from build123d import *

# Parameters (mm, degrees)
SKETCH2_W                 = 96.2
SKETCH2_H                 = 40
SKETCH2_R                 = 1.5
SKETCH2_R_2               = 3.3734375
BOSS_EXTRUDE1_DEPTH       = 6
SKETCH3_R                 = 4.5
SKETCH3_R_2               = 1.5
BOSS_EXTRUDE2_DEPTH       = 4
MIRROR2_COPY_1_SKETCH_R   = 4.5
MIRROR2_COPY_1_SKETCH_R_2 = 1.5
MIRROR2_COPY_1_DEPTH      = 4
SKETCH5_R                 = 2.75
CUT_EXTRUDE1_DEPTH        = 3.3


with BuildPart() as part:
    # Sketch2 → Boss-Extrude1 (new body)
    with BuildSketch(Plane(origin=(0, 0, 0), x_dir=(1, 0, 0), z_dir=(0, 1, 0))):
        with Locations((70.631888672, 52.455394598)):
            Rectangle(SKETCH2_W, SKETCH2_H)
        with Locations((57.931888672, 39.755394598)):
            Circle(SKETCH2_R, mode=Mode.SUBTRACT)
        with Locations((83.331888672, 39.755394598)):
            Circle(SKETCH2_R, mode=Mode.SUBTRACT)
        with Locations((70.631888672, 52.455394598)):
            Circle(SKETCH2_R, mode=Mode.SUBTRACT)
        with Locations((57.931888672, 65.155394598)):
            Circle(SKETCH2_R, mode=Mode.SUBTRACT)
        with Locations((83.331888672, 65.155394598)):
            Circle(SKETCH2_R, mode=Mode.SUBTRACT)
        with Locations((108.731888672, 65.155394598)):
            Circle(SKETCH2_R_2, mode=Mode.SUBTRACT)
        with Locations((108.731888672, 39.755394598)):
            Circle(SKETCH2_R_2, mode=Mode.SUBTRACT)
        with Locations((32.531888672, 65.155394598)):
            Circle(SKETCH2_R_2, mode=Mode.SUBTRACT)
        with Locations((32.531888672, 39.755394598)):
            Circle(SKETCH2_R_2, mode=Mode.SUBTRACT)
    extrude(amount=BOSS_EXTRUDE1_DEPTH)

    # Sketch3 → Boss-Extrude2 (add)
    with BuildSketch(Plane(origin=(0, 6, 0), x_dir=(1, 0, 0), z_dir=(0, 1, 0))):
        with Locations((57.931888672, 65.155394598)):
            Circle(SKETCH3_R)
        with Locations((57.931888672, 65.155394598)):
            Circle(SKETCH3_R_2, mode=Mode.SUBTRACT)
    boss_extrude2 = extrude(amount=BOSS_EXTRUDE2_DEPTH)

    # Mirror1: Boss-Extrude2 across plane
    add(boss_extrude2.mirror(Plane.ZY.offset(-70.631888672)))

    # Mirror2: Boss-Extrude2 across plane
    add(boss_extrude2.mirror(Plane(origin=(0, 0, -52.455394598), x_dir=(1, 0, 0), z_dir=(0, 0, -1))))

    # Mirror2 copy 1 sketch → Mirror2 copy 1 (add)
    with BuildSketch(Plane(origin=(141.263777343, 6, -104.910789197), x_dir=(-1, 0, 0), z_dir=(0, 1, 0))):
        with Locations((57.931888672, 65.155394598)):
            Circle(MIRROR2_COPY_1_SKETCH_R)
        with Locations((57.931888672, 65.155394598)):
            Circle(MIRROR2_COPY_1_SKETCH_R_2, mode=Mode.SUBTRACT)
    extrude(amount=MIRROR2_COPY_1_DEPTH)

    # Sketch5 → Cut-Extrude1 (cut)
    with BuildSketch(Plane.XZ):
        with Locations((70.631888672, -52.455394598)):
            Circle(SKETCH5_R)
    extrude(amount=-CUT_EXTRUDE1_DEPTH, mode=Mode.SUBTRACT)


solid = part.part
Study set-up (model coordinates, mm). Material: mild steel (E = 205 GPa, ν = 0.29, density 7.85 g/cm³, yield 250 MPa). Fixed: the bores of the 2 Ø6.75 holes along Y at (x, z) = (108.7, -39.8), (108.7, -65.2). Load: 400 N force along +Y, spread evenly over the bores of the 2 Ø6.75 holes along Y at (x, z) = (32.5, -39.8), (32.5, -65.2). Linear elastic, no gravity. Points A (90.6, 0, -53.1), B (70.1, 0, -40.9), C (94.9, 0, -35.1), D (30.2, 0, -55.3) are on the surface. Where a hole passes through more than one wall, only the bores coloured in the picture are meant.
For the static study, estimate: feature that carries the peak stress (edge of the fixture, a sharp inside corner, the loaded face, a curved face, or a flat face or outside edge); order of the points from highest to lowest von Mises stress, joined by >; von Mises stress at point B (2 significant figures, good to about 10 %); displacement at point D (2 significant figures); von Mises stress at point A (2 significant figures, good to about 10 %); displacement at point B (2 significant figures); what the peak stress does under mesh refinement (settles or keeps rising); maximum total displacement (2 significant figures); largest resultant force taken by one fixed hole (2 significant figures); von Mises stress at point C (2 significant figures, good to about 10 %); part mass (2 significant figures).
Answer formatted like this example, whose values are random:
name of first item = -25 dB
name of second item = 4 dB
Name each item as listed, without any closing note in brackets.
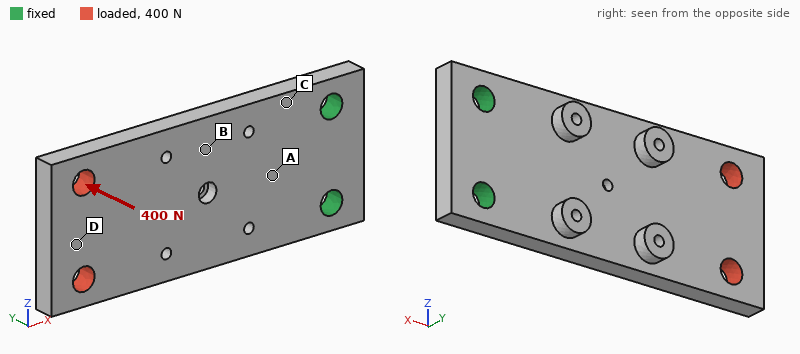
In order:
feature that carries the peak stress = edge of the fixture
order of the points from highest to lowest von Mises stress, joined by > = C > A > B > D
von Mises stress at point B = 64 MPa
displacement at point D = 0.39 mm
von Mises stress at point A = 89 MPa
displacement at point B = 0.12 mm
what the peak stress does under mesh refinement = keeps rising
maximum total displacement = 0.45 mm
largest resultant force taken by one fixed hole = 200 N
von Mises stress at point C = 110 MPa
part mass = 180 g
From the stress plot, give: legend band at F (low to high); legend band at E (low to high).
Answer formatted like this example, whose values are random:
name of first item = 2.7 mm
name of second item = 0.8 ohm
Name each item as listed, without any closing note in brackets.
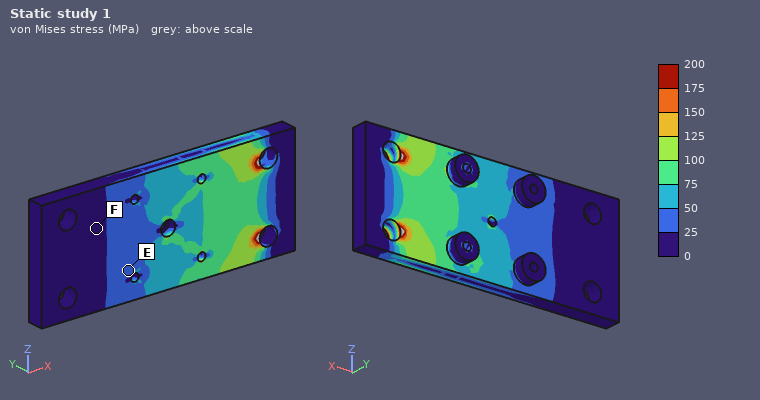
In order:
legend band at F = 0 to 25 MPa
legend band at E = 25 to 50 MPa
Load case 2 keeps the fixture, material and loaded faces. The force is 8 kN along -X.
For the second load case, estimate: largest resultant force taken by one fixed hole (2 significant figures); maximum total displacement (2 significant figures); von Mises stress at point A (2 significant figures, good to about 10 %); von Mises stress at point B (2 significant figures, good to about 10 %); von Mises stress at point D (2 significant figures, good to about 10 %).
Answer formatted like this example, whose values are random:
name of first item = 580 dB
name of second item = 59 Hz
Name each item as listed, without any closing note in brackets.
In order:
largest resultant force taken by one fixed hole = 4.0 kN
maximum total displacement = 18 µm
von Mises stress at point A = 31 MPa
von Mises stress at point B = 35 MPa
von Mises stress at point D = 12 MPa
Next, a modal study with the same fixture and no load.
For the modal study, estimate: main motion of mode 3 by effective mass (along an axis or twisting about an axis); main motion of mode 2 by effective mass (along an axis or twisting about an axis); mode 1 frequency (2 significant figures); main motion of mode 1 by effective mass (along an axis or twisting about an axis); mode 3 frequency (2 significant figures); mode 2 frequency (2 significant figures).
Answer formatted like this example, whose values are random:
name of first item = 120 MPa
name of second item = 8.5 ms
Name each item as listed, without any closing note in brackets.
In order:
main motion of mode 3 by effective mass = along Z
main motion of mode 2 by effective mass = twisting about X
mode 1 frequency = 710 Hz
main motion of mode 1 by effective mass = along Y
mode 3 frequency = 3900 Hz
mode 2 frequency = 3100 Hz
